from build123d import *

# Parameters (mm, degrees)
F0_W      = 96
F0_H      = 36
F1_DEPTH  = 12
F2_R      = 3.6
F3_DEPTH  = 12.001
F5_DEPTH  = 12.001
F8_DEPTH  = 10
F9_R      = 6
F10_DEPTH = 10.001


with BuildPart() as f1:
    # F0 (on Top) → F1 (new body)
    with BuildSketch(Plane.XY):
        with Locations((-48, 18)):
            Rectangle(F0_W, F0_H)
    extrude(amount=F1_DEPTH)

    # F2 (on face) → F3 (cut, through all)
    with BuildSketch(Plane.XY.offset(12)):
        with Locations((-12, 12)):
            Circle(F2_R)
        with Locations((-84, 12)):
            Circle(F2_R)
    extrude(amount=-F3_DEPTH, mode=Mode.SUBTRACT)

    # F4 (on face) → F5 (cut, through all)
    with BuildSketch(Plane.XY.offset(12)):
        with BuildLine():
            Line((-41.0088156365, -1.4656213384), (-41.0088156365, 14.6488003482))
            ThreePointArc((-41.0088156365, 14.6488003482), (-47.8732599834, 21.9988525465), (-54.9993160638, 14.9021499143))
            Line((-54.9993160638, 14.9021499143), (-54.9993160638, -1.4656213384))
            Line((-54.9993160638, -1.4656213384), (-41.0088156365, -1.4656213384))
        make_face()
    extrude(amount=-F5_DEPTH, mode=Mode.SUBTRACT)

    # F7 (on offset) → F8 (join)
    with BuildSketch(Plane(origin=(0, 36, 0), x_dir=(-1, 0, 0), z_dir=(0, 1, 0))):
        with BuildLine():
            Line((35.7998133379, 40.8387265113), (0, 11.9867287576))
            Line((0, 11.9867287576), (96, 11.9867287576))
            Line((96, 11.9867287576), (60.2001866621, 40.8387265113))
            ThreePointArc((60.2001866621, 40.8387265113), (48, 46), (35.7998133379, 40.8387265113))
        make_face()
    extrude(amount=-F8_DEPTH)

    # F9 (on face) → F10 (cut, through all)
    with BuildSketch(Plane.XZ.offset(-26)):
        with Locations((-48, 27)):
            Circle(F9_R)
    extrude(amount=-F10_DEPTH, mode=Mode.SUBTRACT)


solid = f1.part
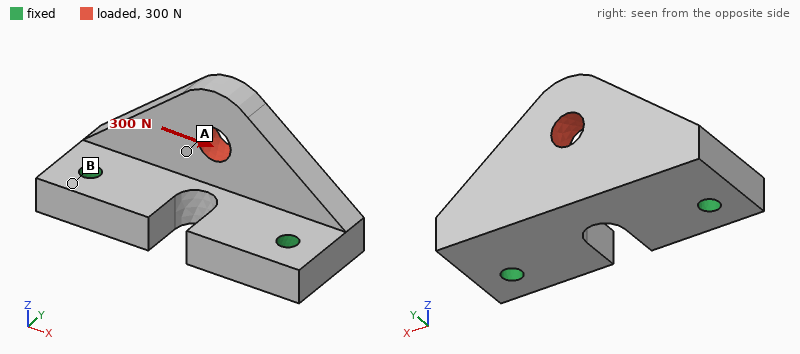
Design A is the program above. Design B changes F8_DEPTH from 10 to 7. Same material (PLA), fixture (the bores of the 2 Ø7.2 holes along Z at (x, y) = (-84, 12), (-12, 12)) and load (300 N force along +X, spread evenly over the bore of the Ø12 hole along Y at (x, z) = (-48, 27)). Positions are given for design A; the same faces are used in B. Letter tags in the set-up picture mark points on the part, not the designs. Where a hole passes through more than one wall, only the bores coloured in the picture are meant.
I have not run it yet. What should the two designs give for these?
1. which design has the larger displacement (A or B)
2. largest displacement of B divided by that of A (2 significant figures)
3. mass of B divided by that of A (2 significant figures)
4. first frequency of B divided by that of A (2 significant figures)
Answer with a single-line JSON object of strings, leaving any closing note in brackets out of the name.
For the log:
{"which design has the larger displacement": "B", "largest displacement of B divided by that of A": "1.3", "mass of B divided by that of A": "0.91", "first frequency of B divided by that of A": "0.98"}
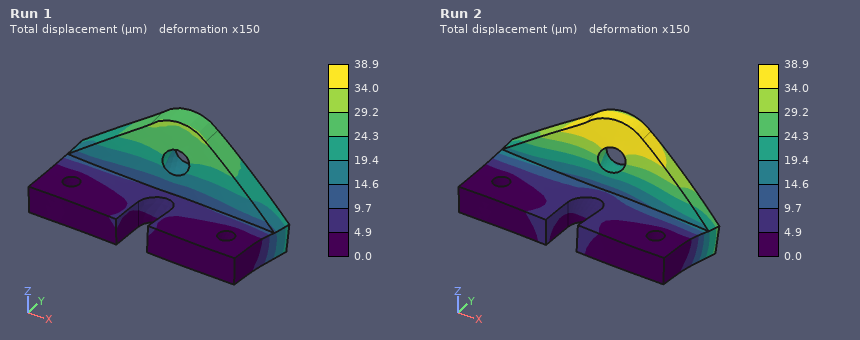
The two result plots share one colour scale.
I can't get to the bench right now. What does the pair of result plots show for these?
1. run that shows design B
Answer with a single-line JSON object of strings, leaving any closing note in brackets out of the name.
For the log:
{"run that shows design B": "Run 2"}
